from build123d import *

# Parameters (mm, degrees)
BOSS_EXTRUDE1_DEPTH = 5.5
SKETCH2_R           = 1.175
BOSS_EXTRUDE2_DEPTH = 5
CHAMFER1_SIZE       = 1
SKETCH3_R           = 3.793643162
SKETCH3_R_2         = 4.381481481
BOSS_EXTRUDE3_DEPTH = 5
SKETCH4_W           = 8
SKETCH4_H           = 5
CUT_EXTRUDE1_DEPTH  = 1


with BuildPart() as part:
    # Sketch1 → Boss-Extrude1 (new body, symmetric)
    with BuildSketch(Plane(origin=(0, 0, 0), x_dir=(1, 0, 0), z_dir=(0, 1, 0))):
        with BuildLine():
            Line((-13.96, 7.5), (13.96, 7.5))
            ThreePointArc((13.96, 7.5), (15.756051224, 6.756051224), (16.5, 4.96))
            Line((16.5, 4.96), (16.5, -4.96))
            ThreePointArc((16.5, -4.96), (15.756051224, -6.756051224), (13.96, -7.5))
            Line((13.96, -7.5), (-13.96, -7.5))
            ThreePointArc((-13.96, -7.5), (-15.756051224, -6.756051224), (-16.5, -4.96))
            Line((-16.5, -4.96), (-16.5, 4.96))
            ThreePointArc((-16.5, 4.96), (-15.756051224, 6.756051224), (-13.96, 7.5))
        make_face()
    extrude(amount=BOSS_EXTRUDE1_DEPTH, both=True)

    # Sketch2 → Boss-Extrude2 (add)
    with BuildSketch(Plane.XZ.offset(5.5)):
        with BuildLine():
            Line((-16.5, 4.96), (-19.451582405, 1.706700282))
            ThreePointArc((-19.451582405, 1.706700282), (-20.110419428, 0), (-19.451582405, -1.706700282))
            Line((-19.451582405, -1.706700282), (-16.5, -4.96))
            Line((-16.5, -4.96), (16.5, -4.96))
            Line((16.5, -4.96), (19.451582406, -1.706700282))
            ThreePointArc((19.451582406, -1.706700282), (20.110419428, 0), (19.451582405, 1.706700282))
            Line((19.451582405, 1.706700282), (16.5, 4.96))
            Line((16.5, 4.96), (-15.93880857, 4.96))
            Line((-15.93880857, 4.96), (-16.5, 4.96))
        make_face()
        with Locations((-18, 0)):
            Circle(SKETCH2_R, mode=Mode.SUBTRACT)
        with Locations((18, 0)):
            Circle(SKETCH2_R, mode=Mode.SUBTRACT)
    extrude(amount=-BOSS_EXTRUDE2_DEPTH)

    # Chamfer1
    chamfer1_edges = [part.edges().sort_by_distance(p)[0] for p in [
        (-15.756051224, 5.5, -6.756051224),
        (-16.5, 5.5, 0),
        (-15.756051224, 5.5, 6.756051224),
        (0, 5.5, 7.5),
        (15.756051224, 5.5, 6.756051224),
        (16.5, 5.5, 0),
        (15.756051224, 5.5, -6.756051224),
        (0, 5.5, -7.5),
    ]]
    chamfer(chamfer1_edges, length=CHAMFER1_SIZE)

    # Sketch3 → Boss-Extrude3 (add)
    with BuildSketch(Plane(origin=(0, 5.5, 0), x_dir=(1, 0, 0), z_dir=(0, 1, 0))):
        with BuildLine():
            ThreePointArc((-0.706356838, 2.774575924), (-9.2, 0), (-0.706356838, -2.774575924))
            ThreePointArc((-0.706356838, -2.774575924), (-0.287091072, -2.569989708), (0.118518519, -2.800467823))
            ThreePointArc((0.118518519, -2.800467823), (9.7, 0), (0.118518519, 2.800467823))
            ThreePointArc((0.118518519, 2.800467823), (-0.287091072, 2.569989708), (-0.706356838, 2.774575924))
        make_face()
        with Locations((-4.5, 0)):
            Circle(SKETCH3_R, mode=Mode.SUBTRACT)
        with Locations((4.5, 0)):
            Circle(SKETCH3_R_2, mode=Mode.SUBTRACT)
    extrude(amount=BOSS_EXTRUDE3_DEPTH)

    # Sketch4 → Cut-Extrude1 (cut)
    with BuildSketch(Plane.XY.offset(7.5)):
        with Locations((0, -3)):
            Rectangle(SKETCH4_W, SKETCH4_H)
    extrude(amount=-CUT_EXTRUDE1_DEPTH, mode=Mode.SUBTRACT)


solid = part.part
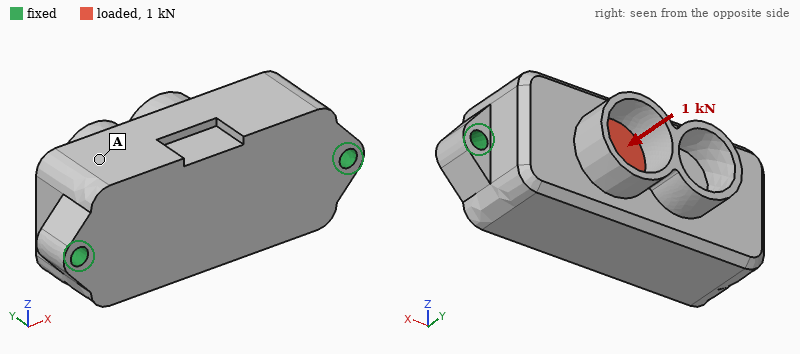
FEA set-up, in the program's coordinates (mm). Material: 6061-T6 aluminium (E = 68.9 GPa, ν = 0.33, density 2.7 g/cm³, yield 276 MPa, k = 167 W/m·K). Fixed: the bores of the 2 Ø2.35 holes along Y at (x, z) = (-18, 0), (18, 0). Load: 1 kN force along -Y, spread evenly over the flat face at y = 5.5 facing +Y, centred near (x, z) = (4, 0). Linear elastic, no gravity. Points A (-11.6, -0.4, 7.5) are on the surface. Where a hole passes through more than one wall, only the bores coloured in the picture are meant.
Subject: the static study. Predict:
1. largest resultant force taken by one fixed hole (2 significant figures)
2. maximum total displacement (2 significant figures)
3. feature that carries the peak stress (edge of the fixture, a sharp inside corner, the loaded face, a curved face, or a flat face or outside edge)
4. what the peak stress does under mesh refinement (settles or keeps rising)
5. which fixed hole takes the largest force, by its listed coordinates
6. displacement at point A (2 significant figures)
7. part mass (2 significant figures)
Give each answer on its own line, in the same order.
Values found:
740 N
7.7 µm
edge of the fixture
keeps rising
(18, 0)
3.2 µm
15 g
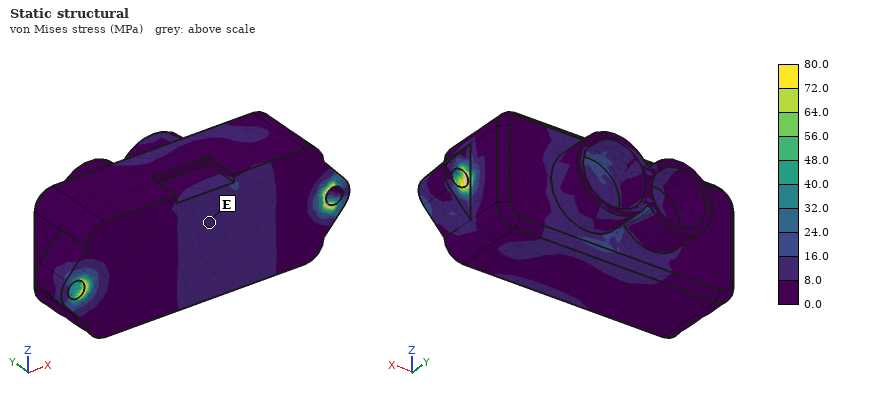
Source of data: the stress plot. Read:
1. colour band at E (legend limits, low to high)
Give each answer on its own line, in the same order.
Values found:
8.0 to 16.0 MPa
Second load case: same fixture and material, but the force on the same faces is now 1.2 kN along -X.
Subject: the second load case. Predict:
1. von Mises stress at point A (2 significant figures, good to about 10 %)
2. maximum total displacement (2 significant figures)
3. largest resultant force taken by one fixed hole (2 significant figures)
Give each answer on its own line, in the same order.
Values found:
4.7 MPa
4.6 µm
680 N
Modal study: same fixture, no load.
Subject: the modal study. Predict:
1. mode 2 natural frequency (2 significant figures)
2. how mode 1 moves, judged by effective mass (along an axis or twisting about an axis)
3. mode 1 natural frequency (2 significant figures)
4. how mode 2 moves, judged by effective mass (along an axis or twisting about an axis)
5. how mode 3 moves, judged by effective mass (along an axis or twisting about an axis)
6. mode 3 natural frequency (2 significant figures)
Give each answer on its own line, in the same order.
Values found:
19 kHz
along Z
12 kHz
along Y
along Z
24 kHz
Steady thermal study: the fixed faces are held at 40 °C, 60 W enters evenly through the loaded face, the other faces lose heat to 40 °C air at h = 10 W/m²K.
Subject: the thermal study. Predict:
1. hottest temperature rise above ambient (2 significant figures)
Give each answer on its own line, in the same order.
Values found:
45 K
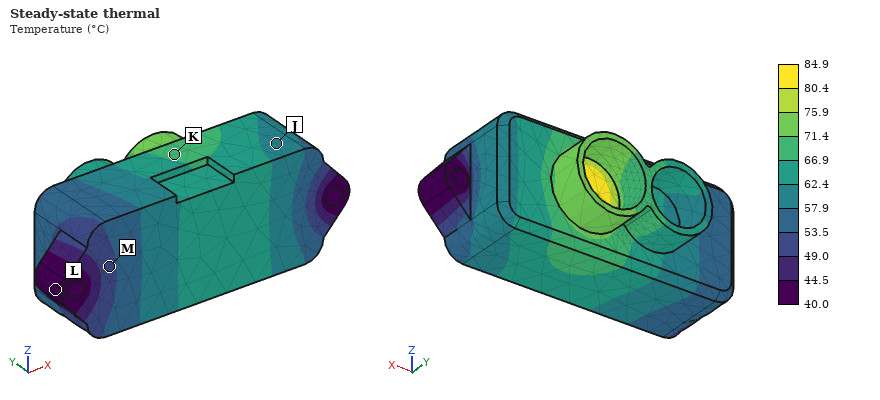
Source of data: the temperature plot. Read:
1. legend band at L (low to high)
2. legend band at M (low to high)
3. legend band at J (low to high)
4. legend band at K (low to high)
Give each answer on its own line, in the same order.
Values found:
40.0 to 44.5 °C
49.0 to 53.5 °C
57.9 to 62.4 °C
66.9 to 71.4 °C
